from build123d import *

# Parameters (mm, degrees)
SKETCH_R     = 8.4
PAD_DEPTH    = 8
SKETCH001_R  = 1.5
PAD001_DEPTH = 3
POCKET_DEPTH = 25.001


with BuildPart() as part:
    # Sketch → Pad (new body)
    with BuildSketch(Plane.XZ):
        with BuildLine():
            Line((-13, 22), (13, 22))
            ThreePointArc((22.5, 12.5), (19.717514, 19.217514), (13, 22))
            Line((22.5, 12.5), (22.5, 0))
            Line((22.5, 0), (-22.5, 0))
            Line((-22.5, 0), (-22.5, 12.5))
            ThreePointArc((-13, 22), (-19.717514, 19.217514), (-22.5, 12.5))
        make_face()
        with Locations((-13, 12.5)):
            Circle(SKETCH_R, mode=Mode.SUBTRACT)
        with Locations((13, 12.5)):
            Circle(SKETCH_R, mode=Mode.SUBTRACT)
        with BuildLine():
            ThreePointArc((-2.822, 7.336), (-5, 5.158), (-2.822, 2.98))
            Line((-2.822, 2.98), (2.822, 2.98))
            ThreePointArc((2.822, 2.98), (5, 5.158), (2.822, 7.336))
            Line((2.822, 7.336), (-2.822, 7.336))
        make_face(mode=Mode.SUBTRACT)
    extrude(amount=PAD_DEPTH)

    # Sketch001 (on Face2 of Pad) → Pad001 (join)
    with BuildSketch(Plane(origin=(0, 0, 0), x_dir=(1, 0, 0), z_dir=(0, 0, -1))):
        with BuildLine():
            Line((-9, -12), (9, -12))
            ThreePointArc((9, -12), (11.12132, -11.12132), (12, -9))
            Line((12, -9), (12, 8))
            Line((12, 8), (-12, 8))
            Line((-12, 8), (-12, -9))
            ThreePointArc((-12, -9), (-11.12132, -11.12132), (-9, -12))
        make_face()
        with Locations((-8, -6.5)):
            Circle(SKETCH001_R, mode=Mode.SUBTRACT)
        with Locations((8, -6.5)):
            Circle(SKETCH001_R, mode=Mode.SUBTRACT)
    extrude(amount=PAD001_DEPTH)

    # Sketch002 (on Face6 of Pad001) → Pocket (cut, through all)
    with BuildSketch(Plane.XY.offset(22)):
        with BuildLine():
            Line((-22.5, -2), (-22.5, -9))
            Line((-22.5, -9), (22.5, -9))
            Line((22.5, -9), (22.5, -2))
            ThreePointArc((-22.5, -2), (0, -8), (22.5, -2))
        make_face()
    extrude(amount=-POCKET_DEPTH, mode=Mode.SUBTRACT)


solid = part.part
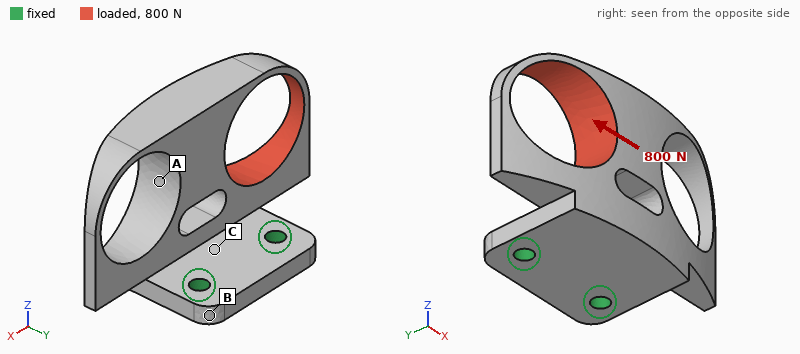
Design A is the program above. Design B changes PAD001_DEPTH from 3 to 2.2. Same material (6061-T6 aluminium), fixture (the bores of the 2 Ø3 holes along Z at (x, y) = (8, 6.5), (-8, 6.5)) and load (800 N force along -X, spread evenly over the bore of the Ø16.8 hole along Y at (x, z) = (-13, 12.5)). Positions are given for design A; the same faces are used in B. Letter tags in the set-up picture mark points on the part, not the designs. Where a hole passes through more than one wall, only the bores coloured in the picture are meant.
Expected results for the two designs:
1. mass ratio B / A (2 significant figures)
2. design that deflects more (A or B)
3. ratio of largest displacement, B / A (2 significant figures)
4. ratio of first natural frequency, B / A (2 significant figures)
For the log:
0.92
B
1.5
0.69
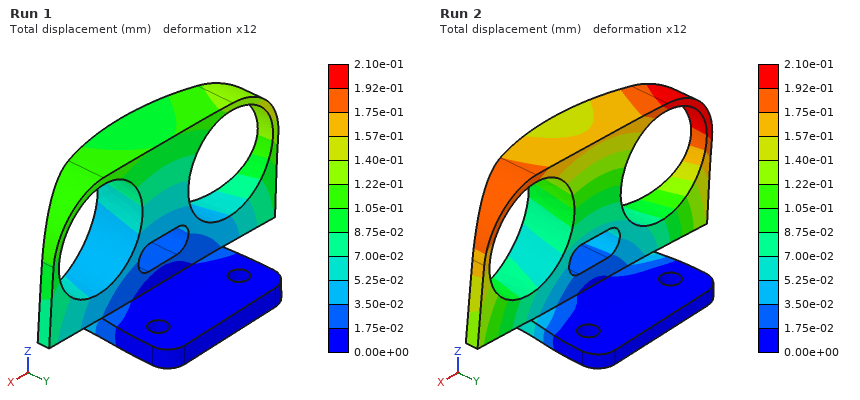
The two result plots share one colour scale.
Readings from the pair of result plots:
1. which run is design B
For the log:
Run 2
